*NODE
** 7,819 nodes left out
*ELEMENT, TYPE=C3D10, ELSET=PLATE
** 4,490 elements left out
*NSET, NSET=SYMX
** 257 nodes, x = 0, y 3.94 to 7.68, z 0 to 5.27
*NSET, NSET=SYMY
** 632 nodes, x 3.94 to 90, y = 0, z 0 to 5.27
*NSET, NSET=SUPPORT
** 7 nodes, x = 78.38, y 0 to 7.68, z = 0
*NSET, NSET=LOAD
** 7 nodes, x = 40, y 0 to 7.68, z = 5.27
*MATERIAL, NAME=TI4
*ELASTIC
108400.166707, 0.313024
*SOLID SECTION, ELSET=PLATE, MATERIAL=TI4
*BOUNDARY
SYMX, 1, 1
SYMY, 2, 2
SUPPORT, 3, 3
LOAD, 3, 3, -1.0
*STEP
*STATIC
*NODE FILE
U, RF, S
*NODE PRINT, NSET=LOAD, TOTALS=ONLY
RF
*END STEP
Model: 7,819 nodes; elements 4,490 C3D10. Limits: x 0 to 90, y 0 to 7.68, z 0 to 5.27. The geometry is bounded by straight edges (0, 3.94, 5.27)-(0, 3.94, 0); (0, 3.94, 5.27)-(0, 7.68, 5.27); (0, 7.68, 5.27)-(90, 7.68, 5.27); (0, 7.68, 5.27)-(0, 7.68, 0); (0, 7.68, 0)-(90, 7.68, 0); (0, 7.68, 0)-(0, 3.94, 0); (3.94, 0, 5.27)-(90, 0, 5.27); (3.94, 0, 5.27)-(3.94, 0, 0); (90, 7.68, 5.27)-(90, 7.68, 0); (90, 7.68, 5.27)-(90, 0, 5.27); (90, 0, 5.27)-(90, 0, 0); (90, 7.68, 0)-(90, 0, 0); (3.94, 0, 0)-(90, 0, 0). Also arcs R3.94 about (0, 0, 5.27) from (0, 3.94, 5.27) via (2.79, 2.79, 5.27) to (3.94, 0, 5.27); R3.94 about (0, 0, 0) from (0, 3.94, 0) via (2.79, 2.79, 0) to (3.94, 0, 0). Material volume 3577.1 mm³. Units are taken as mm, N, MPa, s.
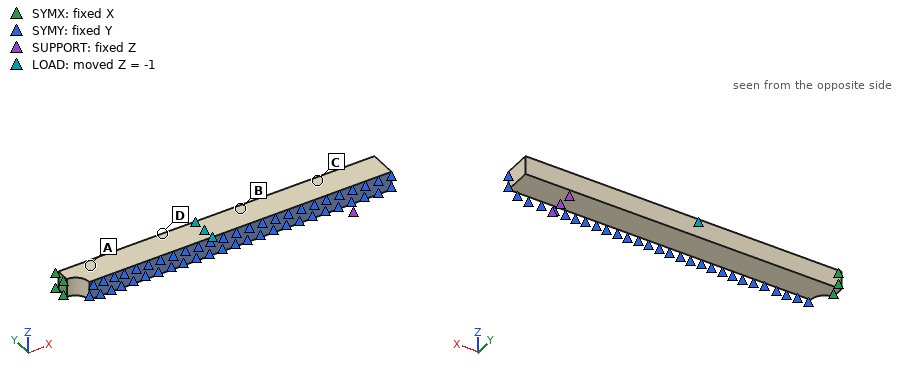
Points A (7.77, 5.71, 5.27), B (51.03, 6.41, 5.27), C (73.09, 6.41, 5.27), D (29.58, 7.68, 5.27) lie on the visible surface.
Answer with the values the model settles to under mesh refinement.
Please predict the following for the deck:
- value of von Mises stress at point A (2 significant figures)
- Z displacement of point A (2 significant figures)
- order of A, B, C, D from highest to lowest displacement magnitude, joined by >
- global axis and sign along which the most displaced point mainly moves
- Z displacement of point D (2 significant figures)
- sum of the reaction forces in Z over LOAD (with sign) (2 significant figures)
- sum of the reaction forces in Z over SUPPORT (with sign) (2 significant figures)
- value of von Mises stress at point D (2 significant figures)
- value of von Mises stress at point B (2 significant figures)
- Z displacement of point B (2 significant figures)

150 MPa
-1.4 mm
A > D > B > C
-Z
-1.2 mm
-120 N
120 N
130 MPa
93 MPa
-0.75 mm
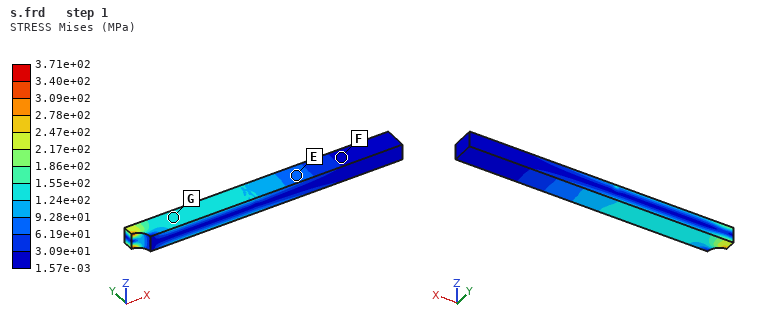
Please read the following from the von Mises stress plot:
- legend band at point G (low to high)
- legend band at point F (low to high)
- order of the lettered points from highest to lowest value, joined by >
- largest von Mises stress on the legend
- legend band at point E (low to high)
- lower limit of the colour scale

1.24e+02 to 1.55e+02 MPa
1.57e-03 to 3.09e+01 MPa
G > E > F
3.71e+02 MPa
6.19e+01 to 9.28e+01 MPa
1.57e-03 MPa
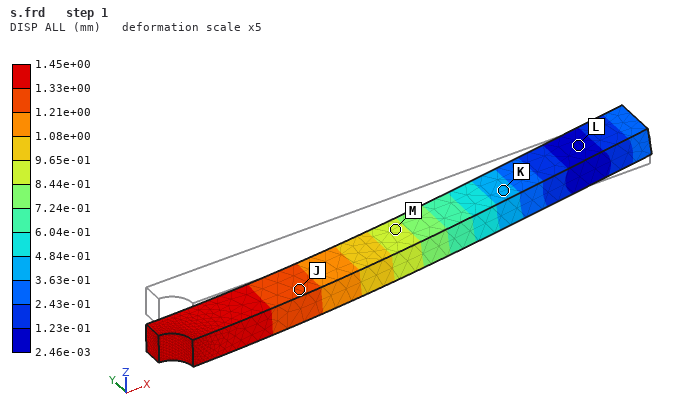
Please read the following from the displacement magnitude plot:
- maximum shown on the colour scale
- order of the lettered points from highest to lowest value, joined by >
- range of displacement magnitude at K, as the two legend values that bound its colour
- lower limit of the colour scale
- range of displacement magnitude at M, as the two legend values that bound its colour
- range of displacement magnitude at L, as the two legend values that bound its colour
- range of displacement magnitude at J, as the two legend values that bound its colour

1.45e+00 mm
J > M > K > L
3.63e-01 to 4.84e-01 mm
2.46e-03 mm
8.44e-01 to 9.65e-01 mm
2.46e-03 to 1.23e-01 mm
1.21e+00 to 1.33e+00 mm
